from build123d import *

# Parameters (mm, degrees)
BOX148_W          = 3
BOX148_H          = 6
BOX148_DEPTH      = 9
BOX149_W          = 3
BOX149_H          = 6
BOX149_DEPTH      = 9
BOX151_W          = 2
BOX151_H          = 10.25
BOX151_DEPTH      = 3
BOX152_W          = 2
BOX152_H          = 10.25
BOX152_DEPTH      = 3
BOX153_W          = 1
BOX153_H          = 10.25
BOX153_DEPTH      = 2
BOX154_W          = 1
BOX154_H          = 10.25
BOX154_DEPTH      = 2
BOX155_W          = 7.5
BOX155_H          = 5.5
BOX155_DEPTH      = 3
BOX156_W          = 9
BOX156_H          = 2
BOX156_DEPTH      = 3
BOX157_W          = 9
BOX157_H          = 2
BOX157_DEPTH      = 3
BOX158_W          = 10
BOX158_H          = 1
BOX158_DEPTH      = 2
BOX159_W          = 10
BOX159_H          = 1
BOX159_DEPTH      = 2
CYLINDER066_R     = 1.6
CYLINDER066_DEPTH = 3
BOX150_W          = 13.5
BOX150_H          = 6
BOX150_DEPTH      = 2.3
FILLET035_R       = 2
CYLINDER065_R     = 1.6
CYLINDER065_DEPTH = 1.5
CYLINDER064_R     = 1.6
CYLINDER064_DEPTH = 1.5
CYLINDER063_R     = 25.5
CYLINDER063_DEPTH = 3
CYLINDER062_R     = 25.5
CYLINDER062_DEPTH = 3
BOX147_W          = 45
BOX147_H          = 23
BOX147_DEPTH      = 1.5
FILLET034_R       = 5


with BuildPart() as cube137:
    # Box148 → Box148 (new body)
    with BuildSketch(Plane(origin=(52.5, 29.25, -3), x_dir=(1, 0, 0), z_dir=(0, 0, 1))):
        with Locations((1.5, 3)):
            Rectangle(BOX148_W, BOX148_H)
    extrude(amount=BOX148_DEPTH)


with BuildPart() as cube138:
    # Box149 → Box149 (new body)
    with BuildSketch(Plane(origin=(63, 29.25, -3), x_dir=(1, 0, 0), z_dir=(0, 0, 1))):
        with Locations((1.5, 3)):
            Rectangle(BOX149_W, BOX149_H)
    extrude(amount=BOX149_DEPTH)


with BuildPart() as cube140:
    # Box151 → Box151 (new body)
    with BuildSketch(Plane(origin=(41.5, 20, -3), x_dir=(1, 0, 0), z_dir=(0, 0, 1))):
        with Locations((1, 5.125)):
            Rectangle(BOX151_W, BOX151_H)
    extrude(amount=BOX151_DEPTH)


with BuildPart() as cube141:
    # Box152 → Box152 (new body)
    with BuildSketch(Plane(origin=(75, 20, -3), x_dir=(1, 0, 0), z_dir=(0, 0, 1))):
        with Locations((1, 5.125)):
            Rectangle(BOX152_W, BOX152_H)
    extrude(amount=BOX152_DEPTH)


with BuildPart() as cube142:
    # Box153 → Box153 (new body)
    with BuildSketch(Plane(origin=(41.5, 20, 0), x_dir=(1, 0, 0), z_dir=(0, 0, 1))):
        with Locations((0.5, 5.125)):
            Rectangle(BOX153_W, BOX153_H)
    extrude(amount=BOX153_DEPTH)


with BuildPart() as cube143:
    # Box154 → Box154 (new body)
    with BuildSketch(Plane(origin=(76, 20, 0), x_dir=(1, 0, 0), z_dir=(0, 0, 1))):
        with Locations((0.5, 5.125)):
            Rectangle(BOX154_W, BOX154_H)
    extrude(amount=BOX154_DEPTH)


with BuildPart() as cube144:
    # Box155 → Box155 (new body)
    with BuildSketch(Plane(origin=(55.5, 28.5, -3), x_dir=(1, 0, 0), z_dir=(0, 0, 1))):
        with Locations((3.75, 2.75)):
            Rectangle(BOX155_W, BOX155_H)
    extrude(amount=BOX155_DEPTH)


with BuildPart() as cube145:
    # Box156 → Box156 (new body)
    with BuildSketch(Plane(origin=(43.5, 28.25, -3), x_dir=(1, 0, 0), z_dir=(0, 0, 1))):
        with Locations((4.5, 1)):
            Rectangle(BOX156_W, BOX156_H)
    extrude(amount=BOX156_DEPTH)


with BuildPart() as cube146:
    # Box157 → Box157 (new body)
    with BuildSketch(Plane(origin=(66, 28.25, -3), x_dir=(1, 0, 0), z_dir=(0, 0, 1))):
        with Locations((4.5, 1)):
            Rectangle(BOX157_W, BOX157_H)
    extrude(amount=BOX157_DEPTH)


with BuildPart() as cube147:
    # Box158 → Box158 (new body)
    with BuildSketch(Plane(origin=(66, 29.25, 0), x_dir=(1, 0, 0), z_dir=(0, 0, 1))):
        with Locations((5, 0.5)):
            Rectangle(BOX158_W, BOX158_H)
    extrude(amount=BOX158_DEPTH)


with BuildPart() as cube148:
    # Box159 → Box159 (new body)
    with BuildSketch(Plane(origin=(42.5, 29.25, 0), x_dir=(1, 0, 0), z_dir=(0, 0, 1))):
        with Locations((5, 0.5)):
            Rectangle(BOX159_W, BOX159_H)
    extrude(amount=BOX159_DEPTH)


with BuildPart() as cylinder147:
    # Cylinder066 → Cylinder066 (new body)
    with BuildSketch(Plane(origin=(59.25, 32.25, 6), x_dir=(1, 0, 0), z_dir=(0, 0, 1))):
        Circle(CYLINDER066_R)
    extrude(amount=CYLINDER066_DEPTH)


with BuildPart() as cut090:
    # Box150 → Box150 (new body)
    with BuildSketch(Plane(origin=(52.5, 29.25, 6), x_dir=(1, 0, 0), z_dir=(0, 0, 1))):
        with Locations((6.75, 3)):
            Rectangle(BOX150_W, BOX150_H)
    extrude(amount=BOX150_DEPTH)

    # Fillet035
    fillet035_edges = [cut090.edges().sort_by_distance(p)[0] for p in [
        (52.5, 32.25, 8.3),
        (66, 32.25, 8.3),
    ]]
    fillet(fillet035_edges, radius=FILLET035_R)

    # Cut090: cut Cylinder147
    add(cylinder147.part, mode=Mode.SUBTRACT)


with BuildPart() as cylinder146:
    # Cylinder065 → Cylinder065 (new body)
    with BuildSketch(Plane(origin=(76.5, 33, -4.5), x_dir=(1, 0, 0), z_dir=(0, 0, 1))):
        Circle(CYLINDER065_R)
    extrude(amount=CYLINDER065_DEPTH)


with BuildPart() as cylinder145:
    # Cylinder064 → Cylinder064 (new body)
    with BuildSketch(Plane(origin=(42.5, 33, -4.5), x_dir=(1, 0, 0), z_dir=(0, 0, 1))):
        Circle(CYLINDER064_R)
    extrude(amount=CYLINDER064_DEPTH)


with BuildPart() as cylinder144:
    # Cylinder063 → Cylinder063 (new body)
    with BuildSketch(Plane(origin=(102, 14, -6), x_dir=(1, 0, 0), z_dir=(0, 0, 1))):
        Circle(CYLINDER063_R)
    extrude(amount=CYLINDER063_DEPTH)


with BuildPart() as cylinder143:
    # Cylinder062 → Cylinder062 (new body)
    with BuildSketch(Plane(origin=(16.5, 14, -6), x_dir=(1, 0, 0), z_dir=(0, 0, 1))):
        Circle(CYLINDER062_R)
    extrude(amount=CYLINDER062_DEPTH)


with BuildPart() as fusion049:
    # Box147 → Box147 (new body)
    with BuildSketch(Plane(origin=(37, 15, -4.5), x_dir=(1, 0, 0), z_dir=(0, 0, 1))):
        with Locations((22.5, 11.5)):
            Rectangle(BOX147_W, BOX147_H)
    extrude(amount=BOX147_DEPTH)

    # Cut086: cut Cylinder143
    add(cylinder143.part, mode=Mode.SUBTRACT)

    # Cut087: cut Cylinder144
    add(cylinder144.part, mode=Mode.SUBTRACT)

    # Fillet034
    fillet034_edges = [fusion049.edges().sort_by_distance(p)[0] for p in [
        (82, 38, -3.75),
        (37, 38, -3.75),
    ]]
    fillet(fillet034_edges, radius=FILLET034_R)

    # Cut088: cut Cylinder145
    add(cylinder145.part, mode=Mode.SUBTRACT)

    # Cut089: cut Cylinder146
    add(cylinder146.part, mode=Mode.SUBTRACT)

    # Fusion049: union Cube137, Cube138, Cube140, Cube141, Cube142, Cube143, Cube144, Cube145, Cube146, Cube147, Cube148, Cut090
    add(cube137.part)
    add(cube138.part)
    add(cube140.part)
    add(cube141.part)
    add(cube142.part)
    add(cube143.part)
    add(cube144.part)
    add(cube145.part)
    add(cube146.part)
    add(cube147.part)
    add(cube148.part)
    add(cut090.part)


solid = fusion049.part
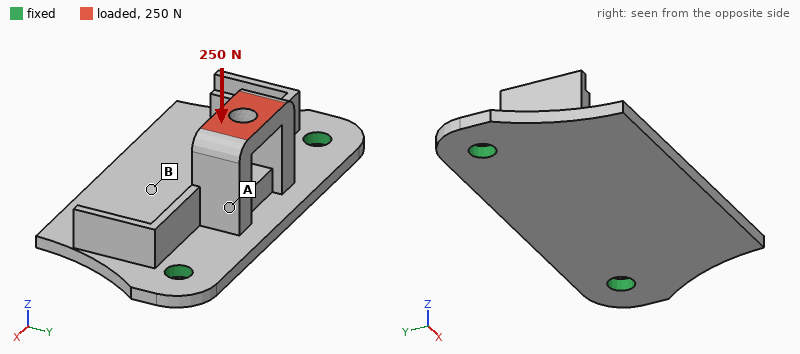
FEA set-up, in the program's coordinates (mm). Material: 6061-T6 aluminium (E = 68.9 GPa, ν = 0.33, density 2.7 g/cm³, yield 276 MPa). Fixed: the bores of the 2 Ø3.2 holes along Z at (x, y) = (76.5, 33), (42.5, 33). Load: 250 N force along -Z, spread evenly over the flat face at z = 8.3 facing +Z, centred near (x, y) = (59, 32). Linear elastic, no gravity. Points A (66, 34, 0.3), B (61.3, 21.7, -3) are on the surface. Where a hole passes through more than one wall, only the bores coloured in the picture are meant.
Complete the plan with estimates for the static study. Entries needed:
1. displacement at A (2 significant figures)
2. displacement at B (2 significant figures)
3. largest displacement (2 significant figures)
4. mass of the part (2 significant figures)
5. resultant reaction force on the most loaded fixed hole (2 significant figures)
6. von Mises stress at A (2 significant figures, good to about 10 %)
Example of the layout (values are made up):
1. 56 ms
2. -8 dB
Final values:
1. 31 µm
2. 7.6 µm
3. 47 µm
4. 6.2 g
5. 160 N
6. 21 MPa
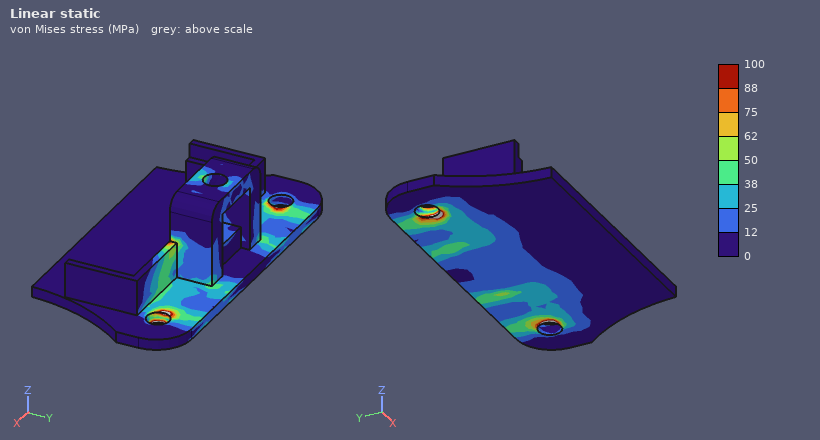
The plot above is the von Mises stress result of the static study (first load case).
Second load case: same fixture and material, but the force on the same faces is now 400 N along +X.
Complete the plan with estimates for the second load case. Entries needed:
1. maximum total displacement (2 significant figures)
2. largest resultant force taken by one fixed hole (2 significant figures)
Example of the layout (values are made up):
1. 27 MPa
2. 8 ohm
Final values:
1. 37 µm
2. 250 N
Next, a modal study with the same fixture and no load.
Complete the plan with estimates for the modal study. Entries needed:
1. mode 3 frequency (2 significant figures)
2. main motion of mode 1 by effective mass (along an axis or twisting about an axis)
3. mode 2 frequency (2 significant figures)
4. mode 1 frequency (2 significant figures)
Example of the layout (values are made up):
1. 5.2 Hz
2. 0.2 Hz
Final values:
1. 7800 Hz
2. along Z
3. 7700 Hz
4. 3600 Hz
